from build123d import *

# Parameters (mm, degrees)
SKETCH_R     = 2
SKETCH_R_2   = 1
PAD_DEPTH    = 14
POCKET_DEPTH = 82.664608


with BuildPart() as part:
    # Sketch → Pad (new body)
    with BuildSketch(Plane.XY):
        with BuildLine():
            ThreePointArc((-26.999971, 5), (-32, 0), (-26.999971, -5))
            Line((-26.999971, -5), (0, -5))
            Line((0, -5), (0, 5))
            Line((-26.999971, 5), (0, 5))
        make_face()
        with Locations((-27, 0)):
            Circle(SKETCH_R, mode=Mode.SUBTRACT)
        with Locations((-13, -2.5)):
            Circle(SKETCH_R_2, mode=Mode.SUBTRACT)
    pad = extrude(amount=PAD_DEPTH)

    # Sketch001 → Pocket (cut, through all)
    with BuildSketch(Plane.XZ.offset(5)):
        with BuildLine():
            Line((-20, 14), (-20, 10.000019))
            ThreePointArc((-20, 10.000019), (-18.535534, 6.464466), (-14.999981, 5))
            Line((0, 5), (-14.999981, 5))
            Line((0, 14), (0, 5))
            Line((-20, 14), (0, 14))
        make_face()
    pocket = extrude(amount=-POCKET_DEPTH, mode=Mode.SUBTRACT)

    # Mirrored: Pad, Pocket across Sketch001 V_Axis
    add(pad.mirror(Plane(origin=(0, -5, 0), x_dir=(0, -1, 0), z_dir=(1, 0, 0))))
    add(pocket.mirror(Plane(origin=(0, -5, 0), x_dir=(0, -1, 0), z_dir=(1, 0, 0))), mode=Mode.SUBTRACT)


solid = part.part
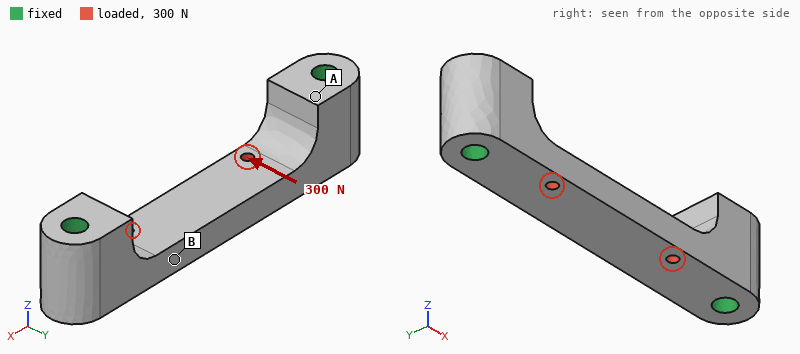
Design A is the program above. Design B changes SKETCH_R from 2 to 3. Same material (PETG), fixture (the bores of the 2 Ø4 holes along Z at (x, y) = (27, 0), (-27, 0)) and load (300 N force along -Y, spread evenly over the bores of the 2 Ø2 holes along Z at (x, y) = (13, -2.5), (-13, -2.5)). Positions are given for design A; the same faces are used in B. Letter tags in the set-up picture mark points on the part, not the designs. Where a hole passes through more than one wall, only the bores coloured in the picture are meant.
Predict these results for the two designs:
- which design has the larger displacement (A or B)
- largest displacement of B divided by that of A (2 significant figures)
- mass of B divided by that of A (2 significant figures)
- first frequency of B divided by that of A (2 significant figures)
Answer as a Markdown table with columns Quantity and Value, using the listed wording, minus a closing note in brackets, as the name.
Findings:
| Quantity | Value |
|---|---|
| which design has the larger displacement | A |
| largest displacement of B divided by that of A | 0.80 |
| mass of B divided by that of A | 0.91 |
| first frequency of B divided by that of A | 1.0 |
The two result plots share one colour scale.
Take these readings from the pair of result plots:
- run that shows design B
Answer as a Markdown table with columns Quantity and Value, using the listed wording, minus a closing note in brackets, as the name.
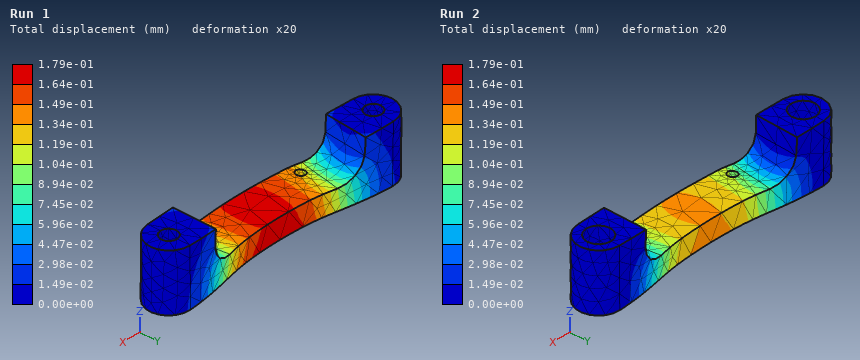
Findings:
| Quantity | Value |
|---|---|
| run that shows design B | Run 2 |
